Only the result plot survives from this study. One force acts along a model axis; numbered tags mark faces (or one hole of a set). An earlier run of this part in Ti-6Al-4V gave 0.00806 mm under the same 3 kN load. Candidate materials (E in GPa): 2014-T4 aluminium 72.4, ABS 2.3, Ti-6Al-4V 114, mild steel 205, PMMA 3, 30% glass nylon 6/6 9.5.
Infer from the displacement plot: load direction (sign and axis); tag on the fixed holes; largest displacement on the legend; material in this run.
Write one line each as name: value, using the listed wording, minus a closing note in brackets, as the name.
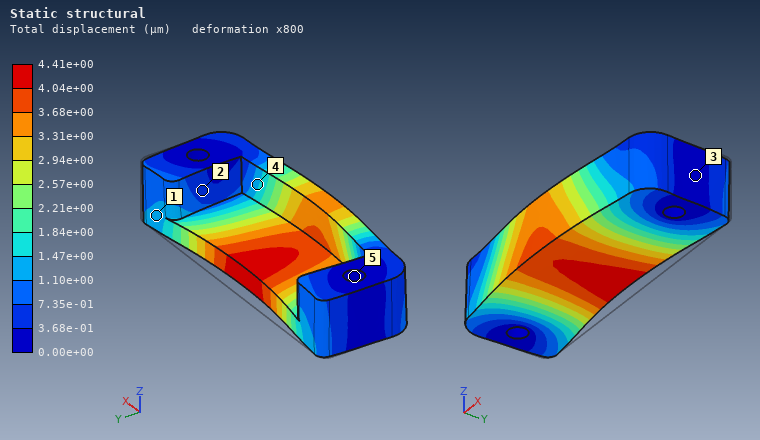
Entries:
load direction: -Y
tag on the fixed holes: 5
largest displacement on the legend: 4.41e+00 µm
material in this run: mild steel
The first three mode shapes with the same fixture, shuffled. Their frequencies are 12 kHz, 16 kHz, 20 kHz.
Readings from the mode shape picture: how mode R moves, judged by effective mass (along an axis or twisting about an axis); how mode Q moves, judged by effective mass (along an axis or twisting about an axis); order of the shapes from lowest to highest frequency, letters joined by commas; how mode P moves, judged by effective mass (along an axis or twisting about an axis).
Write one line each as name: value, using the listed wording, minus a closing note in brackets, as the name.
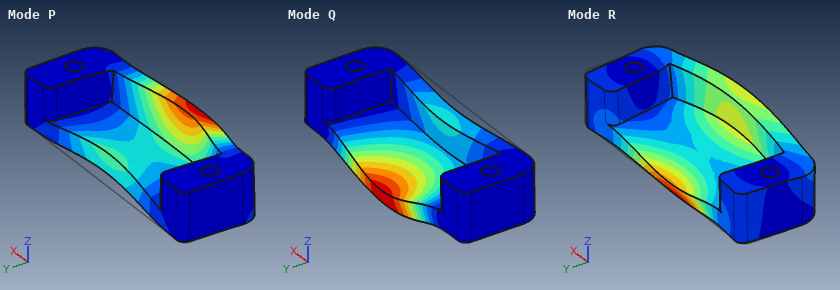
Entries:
how mode R moves, judged by effective mass: along Y
how mode Q moves, judged by effective mass: along Z
order of the shapes from lowest to highest frequency, letters joined by commas: Q, P, R
how mode P moves, judged by effective mass: along Y
